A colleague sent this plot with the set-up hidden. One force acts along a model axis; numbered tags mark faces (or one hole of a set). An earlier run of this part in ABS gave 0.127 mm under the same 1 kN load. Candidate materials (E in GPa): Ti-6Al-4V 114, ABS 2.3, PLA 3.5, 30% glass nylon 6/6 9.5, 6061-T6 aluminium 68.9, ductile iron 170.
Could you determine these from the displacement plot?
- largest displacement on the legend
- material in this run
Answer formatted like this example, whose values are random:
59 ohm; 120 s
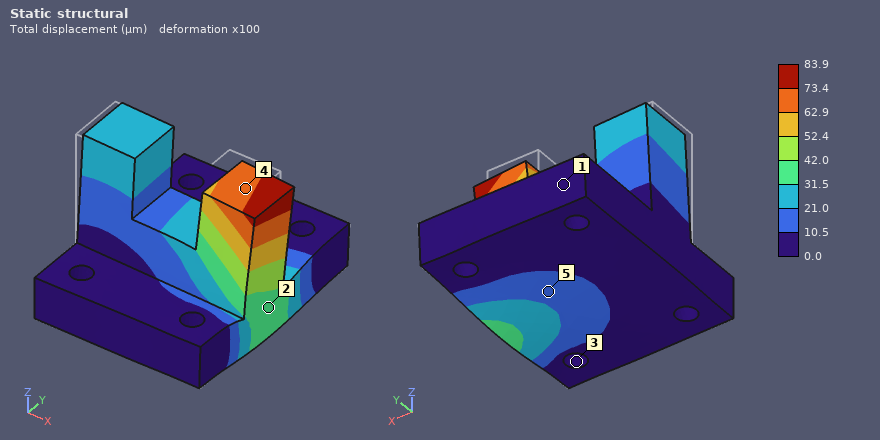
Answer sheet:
83.9 µm; PLA
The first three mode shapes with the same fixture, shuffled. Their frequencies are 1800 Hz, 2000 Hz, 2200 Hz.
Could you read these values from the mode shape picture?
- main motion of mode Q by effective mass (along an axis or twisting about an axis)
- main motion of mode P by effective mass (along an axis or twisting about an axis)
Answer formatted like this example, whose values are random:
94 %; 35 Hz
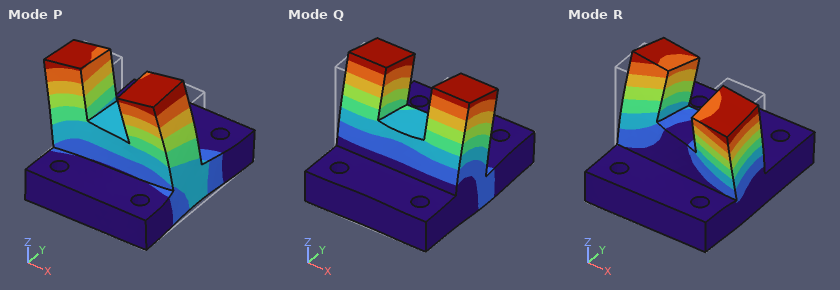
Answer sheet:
along Y; along X
